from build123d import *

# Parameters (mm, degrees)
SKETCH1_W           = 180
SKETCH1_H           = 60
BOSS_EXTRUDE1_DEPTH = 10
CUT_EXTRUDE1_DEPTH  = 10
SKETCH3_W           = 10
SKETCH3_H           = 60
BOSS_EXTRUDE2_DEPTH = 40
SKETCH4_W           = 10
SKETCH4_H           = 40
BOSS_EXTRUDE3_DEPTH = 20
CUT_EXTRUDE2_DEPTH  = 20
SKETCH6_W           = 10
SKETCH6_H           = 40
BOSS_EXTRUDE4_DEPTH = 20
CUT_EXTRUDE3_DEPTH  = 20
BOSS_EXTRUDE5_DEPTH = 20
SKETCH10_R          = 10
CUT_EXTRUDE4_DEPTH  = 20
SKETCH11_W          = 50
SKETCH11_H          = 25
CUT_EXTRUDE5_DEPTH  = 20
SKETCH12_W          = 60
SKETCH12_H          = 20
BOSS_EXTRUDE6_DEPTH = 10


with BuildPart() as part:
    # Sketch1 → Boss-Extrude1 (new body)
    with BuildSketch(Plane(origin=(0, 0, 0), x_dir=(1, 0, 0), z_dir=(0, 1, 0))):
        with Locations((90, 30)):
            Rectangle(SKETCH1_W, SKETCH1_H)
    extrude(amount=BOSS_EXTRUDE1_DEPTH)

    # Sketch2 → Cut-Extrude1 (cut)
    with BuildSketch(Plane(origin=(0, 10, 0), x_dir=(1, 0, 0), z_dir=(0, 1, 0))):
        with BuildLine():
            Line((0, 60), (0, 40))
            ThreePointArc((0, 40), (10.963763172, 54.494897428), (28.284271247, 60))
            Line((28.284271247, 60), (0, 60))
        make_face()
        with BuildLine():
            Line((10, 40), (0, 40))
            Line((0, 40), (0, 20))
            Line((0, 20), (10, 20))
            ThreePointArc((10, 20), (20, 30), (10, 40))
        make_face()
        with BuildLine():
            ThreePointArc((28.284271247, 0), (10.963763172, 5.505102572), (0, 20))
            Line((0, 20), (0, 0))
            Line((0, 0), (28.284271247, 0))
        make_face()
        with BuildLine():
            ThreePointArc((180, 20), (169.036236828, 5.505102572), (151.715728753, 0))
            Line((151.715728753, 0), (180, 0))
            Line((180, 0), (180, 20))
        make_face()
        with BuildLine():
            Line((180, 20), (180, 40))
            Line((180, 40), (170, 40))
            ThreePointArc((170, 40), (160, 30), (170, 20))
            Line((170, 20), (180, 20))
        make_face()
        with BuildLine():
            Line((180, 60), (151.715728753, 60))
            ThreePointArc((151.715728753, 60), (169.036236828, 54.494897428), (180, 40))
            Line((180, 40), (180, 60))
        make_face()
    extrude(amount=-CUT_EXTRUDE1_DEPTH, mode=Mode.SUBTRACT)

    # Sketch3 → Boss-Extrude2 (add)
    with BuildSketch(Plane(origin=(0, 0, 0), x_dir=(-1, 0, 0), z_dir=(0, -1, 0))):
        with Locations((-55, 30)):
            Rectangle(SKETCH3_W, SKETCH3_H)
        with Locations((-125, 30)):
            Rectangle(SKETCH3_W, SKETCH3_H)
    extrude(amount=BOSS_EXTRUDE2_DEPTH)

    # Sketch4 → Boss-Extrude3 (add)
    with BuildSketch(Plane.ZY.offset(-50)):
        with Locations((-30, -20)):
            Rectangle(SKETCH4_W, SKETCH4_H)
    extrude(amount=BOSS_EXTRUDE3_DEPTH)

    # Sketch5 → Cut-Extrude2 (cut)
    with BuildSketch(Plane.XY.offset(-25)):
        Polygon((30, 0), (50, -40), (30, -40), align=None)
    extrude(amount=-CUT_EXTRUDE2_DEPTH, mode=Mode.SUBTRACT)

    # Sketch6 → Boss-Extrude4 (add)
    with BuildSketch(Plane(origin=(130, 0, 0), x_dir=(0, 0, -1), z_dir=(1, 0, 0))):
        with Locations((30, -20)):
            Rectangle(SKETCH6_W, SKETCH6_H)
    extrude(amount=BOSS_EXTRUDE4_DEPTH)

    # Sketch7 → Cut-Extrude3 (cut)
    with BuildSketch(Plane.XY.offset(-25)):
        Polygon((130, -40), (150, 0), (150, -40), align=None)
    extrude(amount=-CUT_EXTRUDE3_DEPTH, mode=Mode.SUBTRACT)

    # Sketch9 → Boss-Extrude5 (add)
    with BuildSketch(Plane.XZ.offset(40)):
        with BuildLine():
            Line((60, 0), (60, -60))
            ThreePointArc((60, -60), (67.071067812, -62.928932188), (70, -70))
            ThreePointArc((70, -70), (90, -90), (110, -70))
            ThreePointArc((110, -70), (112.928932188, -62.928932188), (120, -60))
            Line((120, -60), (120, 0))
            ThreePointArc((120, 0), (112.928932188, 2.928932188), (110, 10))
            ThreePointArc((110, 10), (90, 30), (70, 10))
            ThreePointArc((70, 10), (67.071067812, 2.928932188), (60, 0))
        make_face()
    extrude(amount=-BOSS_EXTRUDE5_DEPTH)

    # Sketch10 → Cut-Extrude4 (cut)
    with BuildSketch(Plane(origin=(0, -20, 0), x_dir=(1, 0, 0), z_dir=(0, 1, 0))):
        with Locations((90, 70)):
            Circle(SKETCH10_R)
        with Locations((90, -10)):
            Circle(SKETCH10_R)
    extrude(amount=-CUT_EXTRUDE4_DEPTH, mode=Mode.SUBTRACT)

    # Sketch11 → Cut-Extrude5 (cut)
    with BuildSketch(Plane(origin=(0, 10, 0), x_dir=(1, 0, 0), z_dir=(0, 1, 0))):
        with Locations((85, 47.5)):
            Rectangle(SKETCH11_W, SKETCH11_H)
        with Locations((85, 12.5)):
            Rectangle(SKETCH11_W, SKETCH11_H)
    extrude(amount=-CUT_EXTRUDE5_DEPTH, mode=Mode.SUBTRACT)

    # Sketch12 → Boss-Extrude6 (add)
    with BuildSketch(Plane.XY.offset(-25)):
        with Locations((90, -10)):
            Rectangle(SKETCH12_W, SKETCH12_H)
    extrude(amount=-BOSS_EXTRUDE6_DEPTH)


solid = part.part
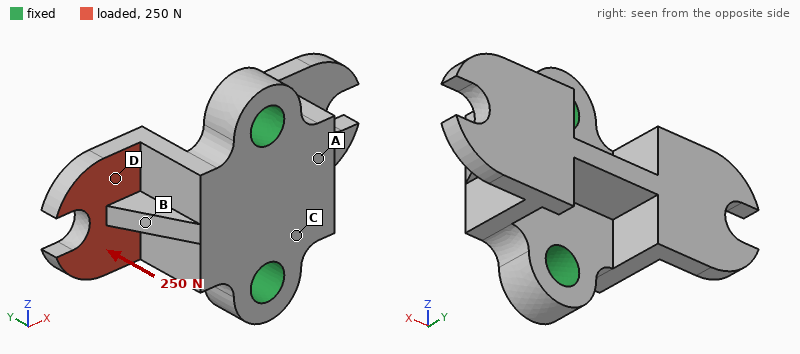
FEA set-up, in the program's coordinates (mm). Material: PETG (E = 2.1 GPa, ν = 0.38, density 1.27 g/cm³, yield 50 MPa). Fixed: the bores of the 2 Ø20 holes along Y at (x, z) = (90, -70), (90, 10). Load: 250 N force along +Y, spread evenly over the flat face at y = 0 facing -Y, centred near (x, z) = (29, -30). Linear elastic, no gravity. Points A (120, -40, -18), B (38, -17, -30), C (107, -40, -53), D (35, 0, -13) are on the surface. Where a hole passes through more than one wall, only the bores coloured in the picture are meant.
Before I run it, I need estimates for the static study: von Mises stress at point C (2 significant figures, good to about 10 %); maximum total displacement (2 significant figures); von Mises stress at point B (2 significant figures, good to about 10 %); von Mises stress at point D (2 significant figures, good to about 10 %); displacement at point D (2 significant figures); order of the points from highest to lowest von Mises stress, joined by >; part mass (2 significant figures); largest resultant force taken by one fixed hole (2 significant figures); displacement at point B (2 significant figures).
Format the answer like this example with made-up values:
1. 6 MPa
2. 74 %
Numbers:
1. 0.62 MPa
2. 0.41 mm
3. 2.3 MPa
4. 1.1 MPa
5. 0.17 mm
6. B > D > C > A
7. 300 g
8. 140 N
9. 0.12 mm
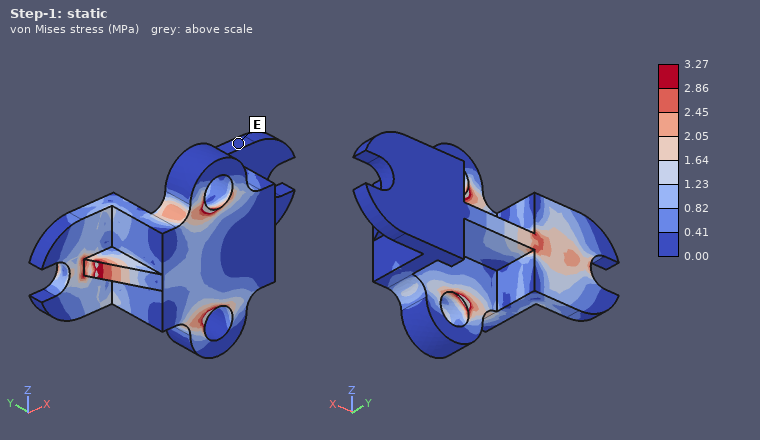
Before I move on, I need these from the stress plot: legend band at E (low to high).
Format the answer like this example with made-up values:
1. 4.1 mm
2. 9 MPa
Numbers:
1. 0.00 to 0.41 MPa
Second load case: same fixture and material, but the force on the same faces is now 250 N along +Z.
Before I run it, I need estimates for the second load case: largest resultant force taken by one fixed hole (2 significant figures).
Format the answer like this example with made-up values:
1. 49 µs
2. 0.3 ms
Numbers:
1. 260 N
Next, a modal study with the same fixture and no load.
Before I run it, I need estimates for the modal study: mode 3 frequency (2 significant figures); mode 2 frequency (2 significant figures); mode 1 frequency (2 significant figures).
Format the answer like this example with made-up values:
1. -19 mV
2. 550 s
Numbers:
1. 1000 Hz
2. 1000 Hz
3. 640 Hz
